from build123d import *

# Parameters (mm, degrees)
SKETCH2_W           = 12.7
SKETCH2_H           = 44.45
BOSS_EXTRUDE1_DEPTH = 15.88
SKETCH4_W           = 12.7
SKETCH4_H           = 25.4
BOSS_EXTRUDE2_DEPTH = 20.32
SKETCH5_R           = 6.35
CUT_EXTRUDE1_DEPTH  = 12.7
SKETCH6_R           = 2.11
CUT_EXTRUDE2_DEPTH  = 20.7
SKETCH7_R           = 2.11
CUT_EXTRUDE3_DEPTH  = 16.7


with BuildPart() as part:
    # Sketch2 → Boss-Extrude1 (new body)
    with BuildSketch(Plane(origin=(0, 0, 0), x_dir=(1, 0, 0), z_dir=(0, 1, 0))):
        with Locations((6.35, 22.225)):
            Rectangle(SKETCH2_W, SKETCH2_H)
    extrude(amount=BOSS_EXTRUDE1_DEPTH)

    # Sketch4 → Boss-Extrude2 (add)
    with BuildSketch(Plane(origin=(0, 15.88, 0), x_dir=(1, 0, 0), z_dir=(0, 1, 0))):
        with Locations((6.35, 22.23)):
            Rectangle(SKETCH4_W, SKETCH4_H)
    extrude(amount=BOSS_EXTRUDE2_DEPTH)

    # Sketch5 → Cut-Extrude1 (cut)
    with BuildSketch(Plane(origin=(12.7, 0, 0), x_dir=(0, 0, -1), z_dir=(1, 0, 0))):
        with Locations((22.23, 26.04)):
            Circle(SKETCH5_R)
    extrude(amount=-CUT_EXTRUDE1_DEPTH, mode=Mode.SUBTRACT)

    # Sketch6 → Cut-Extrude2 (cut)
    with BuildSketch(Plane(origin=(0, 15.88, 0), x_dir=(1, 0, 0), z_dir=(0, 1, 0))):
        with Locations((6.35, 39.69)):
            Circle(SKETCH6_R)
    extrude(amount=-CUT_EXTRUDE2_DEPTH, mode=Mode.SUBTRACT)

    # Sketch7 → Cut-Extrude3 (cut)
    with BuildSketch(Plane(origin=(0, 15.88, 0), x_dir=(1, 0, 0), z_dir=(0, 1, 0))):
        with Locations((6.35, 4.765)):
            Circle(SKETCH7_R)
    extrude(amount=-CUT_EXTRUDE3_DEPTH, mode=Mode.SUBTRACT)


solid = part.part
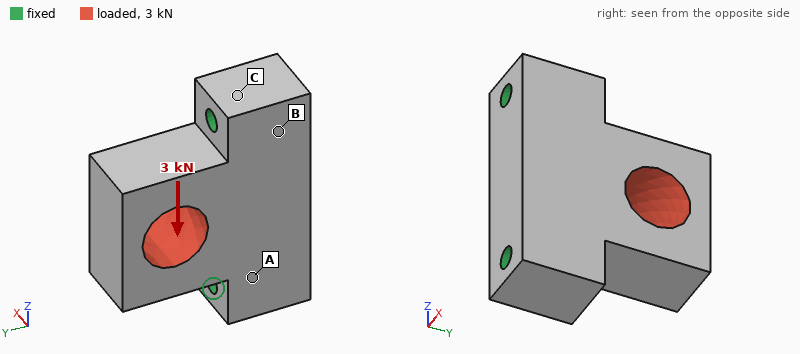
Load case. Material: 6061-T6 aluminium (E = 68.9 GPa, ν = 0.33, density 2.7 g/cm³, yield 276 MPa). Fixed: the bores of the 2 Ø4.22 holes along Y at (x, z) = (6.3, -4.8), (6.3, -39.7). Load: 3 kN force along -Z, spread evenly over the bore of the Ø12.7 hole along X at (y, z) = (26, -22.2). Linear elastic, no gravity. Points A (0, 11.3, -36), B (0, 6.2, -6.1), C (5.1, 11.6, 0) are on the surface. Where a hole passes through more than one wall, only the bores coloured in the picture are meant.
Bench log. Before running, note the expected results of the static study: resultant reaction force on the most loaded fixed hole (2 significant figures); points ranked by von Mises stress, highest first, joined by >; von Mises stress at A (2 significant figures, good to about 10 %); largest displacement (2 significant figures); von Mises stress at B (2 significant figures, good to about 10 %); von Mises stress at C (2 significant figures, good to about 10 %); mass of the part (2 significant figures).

2.1 kN
A > B > C
18 MPa
27 µm
8.9 MPa
5.0 MPa
36 g
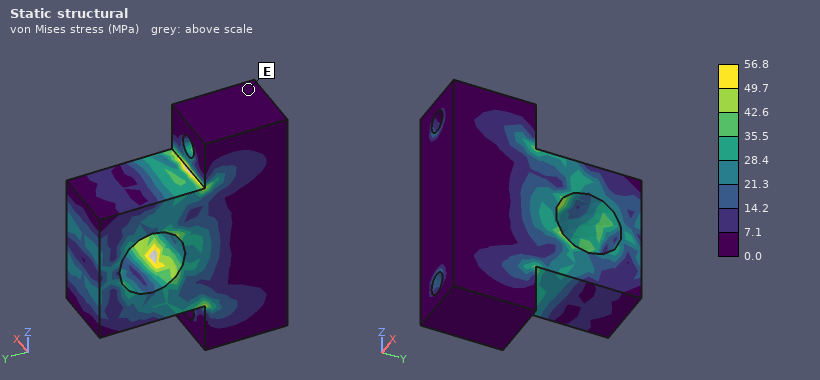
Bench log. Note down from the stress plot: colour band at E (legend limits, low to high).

0.0 to 7.1 MPa
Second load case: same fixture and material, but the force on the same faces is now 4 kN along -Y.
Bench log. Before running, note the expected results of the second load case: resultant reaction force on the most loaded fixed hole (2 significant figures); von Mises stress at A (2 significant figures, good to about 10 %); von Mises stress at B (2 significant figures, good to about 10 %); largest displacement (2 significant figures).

2.1 kN
19 MPa
9.0 MPa
12 µm
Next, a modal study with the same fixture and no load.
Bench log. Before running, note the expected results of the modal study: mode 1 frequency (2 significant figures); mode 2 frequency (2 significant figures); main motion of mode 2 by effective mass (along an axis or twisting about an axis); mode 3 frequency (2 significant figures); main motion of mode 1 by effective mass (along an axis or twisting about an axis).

9700 Hz
17 kHz
along Z
20 kHz
along X
